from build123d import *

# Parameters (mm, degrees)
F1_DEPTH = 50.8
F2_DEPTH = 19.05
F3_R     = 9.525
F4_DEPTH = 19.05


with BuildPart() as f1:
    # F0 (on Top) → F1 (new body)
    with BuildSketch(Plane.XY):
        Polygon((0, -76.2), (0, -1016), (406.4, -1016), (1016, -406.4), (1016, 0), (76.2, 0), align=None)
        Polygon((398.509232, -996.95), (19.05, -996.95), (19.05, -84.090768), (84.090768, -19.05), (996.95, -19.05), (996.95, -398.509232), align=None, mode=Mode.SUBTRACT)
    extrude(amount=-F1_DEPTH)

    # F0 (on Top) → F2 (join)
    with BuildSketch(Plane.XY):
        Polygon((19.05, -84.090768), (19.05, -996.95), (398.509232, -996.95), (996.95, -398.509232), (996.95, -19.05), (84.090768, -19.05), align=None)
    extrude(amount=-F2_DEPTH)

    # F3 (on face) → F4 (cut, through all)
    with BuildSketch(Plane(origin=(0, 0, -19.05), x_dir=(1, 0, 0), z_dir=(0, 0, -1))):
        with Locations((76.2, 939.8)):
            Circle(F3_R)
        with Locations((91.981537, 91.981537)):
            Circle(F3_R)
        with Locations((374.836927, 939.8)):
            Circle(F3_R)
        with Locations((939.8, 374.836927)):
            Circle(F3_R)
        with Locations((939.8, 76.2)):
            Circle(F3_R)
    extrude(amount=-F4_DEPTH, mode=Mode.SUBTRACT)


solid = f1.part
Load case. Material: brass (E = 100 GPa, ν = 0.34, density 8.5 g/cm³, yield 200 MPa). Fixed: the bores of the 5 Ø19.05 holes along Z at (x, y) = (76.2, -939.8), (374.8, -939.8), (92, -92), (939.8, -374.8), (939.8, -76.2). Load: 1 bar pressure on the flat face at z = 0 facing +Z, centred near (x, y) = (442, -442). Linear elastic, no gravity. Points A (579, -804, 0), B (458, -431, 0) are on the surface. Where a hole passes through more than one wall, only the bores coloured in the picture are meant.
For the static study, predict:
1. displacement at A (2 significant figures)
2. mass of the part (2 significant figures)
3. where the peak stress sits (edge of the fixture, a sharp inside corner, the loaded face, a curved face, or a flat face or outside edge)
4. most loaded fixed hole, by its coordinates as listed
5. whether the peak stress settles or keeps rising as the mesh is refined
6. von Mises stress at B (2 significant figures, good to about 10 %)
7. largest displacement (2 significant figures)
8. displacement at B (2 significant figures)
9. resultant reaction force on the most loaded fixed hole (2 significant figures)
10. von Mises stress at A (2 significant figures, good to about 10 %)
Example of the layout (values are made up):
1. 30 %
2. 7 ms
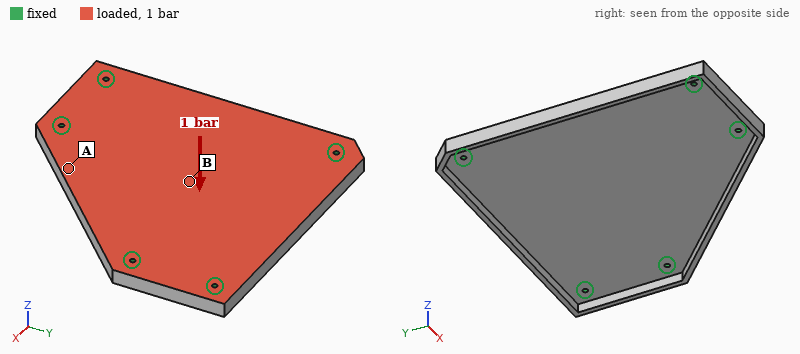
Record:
1. 0.85 mm
2. 150 kg
3. edge of the fixture
4. (92, -92)
5. keeps rising
6. 48 MPa
7. 3.0 mm
8. 3.0 mm
9. 25 kN
10. 21 MPa
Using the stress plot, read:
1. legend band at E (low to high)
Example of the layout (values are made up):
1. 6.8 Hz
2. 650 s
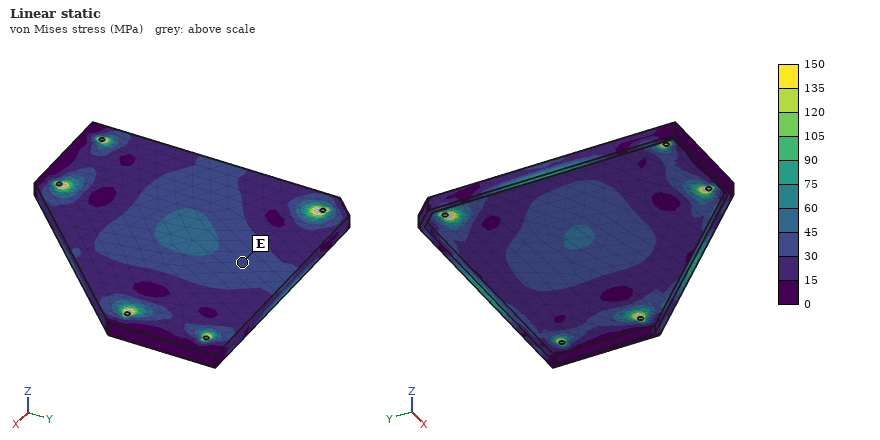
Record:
1. 30 to 45 MPa
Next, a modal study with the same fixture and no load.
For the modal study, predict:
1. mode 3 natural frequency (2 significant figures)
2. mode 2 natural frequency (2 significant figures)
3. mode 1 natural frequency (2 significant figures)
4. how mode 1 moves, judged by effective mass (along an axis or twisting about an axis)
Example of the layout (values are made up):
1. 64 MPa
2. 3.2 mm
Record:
1. 160 Hz
2. 130 Hz
3. 88 Hz
4. along Z
